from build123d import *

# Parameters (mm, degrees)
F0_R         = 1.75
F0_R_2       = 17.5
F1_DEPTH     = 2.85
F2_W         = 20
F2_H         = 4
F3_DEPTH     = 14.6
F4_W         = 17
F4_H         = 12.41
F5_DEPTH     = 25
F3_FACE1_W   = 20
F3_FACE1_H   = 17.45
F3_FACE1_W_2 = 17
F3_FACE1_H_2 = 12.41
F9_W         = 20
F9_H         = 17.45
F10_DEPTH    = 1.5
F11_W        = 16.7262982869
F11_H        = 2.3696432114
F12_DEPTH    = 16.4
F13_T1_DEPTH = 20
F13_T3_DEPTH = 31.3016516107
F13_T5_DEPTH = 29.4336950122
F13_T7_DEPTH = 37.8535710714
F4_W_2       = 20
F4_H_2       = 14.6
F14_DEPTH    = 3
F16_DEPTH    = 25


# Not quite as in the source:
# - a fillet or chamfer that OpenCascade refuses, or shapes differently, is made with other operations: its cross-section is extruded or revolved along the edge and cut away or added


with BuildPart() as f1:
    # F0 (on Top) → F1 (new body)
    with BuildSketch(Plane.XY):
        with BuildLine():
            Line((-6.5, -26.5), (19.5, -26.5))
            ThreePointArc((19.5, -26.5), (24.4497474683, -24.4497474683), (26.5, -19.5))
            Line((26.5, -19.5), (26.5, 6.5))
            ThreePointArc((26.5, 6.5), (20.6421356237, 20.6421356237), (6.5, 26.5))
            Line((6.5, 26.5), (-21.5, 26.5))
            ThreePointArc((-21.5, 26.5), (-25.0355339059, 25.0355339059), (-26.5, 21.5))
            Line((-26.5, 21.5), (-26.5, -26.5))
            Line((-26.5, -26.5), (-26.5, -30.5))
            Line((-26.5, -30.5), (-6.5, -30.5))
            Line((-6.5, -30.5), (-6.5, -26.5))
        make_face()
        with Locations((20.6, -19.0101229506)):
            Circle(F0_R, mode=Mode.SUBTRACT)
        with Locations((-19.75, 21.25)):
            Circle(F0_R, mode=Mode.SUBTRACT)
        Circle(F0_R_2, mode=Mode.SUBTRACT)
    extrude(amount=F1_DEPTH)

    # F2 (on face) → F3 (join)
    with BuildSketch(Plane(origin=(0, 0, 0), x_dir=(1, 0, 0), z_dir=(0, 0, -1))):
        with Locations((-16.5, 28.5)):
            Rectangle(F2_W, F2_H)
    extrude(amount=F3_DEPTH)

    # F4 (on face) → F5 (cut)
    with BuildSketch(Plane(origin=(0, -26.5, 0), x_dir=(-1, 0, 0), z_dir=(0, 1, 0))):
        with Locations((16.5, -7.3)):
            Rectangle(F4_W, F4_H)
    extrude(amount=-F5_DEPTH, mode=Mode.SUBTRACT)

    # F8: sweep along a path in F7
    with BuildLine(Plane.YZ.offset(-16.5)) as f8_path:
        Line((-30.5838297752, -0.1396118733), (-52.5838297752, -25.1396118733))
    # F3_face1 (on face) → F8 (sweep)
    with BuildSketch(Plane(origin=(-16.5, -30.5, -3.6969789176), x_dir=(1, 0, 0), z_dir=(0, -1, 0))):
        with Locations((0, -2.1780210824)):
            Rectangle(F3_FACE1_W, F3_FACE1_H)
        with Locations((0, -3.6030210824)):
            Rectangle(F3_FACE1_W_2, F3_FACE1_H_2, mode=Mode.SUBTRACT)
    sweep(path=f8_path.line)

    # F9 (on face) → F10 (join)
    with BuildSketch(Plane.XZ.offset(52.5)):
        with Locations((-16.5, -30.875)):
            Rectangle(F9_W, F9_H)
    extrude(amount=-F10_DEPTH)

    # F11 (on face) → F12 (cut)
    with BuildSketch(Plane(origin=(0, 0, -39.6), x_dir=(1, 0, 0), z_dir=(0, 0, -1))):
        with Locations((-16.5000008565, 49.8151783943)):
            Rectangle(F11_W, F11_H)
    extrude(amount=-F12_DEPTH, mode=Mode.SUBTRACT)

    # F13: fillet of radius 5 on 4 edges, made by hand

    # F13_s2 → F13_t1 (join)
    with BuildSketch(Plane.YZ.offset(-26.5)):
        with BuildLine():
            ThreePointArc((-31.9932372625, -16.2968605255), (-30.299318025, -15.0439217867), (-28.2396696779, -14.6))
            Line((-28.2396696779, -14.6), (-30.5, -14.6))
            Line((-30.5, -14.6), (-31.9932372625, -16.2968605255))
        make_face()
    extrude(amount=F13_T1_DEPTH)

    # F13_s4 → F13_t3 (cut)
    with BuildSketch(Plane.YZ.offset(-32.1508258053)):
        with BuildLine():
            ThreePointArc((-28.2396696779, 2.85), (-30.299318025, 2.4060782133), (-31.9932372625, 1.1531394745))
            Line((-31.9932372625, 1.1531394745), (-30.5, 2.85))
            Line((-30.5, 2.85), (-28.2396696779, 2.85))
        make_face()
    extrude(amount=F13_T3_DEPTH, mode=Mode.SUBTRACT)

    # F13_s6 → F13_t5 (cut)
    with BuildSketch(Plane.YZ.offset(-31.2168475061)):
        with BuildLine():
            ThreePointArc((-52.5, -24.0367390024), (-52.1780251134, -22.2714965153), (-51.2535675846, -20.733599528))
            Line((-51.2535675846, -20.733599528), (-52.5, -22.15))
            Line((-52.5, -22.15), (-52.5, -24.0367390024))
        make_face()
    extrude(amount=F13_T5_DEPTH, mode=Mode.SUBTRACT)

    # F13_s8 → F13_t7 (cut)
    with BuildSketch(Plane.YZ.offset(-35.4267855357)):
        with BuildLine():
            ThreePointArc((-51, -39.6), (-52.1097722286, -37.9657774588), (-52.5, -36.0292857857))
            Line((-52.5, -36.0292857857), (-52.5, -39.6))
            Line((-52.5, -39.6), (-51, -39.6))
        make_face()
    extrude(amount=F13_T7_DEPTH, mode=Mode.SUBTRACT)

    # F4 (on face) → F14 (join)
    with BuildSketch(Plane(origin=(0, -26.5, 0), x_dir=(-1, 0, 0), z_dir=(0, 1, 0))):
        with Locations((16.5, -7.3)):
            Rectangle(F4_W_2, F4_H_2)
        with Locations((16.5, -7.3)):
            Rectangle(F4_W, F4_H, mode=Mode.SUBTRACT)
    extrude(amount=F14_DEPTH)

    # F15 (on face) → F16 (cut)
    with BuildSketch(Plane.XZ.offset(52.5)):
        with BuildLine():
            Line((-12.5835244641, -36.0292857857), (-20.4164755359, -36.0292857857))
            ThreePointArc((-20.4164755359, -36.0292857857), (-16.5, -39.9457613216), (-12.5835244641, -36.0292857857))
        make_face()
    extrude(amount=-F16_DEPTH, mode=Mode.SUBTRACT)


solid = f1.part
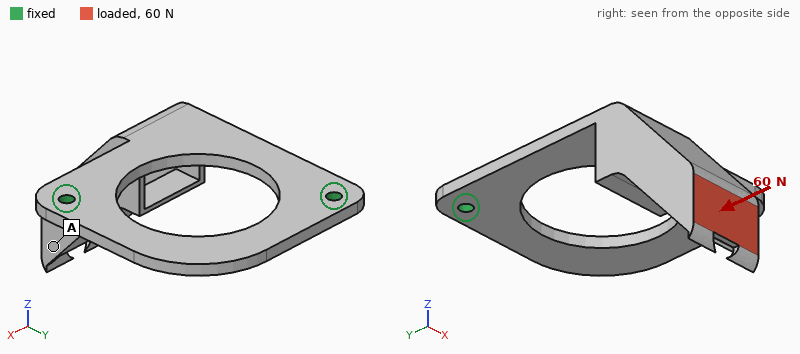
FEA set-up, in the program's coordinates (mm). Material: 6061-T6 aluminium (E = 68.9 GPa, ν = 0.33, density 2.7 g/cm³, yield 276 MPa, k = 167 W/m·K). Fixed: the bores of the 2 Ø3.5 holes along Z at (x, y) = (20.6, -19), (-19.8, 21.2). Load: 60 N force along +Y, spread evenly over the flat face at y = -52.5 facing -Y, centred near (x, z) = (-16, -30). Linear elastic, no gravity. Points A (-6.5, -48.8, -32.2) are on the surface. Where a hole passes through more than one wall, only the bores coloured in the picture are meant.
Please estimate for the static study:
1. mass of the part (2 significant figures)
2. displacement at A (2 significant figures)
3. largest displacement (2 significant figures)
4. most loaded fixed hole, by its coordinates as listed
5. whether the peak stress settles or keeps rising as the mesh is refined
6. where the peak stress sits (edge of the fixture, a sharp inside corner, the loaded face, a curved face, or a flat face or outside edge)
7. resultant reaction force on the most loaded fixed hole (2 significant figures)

24 g
0.80 mm
1.0 mm
(-19.8, 21.2)
keeps rising
edge of the fixture
59 N
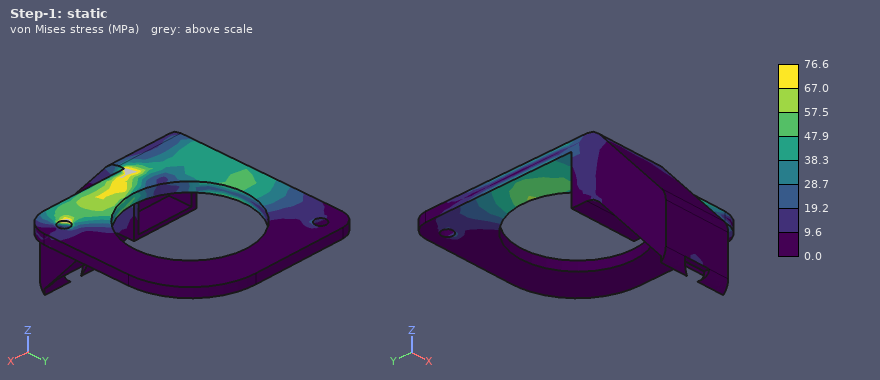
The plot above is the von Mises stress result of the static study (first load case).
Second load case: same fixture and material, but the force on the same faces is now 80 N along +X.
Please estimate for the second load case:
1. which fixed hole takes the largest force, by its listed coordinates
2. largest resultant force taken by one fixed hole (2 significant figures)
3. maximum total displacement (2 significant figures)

(20.6, -19)
120 N
1.1 mm
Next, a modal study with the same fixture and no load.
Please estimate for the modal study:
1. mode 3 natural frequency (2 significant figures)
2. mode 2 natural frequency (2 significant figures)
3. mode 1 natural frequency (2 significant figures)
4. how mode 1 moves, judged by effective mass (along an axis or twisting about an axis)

2000 Hz
1100 Hz
410 Hz
along Z
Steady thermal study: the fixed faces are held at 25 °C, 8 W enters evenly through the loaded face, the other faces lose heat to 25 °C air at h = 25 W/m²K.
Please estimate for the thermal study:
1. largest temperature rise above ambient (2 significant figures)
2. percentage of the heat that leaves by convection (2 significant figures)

38 K
44 %
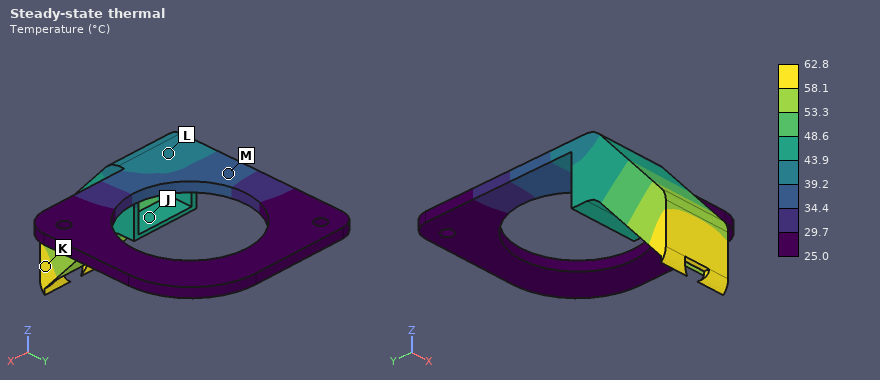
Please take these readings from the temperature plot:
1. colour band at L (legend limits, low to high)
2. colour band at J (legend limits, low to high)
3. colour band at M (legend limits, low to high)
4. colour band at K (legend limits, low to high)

39.2 to 43.9 °C
43.9 to 48.6 °C
34.4 to 39.2 °C
58.1 to 62.8 °C
